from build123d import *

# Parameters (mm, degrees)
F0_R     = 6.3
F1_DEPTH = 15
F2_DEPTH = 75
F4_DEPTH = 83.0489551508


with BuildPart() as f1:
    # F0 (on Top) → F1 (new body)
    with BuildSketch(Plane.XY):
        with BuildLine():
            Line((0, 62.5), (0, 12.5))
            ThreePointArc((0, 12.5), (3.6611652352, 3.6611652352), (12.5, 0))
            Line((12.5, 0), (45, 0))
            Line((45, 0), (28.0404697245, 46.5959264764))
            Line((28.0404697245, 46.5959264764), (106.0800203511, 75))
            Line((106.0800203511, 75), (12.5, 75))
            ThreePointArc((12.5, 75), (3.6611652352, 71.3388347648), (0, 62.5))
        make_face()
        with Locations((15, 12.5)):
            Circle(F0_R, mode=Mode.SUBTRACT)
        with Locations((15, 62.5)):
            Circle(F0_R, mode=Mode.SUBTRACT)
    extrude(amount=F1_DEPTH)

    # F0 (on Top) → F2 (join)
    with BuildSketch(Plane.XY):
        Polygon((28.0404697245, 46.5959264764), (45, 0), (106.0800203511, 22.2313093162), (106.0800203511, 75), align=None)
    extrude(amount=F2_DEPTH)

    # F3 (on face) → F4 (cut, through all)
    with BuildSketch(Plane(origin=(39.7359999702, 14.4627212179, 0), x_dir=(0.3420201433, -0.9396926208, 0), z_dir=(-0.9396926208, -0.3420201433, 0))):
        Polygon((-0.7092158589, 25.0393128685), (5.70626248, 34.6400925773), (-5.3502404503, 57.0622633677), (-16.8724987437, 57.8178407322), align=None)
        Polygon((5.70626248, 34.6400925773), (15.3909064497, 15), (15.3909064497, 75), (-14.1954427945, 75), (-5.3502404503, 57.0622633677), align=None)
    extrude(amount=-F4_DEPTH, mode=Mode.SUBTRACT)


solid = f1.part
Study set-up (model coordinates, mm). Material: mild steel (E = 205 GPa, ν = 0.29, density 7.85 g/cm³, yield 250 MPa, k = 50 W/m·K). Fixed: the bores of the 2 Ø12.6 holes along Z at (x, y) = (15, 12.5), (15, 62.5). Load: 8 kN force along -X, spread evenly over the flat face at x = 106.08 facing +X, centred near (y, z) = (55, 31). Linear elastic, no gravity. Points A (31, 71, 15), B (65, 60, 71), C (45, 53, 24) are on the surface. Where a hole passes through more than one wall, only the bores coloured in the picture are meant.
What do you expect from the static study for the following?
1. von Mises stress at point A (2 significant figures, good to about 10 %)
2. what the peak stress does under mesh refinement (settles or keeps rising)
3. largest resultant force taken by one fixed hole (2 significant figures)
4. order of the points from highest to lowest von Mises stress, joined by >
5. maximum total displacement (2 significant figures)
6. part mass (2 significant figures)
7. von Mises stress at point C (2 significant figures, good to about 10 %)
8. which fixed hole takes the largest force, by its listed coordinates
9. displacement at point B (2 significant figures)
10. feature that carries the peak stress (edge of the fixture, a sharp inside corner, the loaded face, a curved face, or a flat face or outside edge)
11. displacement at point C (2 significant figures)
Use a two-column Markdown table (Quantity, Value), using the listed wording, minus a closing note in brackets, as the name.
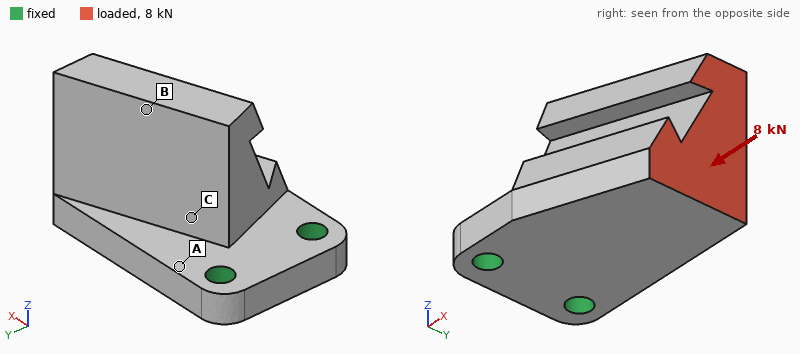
| Quantity | Value |
|---|---|
| von Mises stress at point A | 68 MPa |
| what the peak stress does under mesh refinement | keeps rising |
| largest resultant force taken by one fixed hole | 6.7 kN |
| order of the points from highest to lowest von Mises stress, joined by > | A > C > B |
| maximum total displacement | 0.12 mm |
| part mass | 1.9 kg |
| von Mises stress at point C | 22 MPa |
| which fixed hole takes the largest force, by its listed coordinates | (15, 62.5) |
| displacement at point B | 0.085 mm |
| feature that carries the peak stress | edge of the fixture |
| displacement at point C | 0.027 mm |
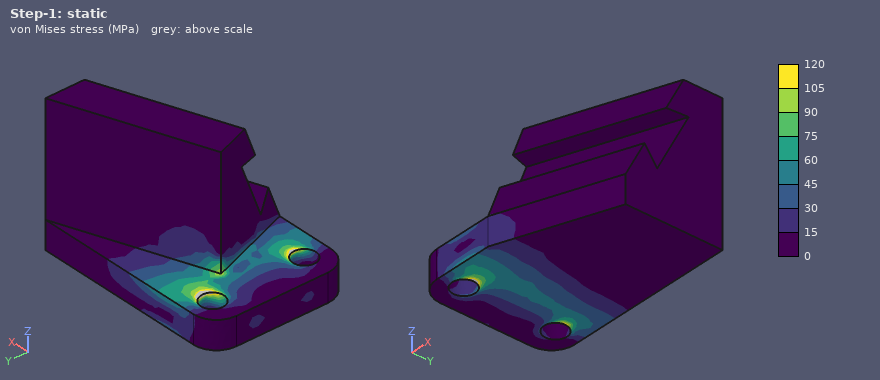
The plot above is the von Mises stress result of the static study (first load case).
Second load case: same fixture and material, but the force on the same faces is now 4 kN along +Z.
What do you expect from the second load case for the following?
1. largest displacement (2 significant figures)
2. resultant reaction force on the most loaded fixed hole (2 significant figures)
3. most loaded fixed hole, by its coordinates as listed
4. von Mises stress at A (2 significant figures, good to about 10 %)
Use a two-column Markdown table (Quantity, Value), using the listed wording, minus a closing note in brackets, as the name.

| Quantity | Value |
|---|---|
| largest displacement | 0.20 mm |
| resultant reaction force on the most loaded fixed hole | 3.3 kN |
| most loaded fixed hole, by its coordinates as listed | (15, 62.5) |
| von Mises stress at A | 100 MPa |
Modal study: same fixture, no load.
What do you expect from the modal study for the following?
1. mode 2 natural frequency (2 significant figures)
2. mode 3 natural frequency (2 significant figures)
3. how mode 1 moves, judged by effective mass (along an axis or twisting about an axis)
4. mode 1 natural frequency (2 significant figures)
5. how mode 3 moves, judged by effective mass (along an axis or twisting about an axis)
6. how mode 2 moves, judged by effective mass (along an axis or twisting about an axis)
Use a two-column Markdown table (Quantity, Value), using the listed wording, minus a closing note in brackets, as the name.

| Quantity | Value |
|---|---|
| mode 2 natural frequency | 2300 Hz |
| mode 3 natural frequency | 4600 Hz |
| how mode 1 moves, judged by effective mass | along Z |
| mode 1 natural frequency | 910 Hz |
| how mode 3 moves, judged by effective mass | along Y |
| how mode 2 moves, judged by effective mass | along Y |
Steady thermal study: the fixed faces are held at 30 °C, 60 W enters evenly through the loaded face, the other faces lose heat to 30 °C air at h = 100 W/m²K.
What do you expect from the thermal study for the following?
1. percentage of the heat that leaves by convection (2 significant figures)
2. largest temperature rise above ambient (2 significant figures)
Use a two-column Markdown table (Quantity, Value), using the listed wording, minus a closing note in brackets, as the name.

| Quantity | Value |
|---|---|
| percentage of the heat that leaves by convection | 69 % |
| largest temperature rise above ambient | 33 K |
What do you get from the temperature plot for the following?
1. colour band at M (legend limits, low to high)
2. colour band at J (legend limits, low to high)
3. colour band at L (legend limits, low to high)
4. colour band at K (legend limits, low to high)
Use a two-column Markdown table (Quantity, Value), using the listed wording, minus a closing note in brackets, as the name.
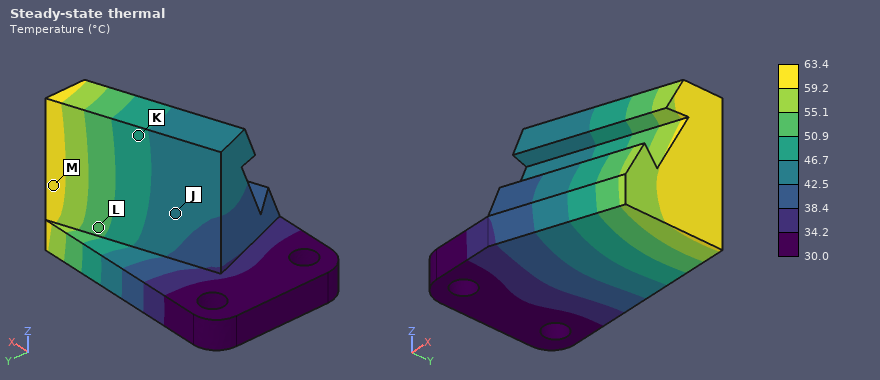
| Quantity | Value |
|---|---|
| colour band at M | 59.2 to 63.4 °C |
| colour band at J | 42.5 to 46.7 °C |
| colour band at L | 50.9 to 55.1 °C |
| colour band at K | 46.7 to 50.9 °C |
